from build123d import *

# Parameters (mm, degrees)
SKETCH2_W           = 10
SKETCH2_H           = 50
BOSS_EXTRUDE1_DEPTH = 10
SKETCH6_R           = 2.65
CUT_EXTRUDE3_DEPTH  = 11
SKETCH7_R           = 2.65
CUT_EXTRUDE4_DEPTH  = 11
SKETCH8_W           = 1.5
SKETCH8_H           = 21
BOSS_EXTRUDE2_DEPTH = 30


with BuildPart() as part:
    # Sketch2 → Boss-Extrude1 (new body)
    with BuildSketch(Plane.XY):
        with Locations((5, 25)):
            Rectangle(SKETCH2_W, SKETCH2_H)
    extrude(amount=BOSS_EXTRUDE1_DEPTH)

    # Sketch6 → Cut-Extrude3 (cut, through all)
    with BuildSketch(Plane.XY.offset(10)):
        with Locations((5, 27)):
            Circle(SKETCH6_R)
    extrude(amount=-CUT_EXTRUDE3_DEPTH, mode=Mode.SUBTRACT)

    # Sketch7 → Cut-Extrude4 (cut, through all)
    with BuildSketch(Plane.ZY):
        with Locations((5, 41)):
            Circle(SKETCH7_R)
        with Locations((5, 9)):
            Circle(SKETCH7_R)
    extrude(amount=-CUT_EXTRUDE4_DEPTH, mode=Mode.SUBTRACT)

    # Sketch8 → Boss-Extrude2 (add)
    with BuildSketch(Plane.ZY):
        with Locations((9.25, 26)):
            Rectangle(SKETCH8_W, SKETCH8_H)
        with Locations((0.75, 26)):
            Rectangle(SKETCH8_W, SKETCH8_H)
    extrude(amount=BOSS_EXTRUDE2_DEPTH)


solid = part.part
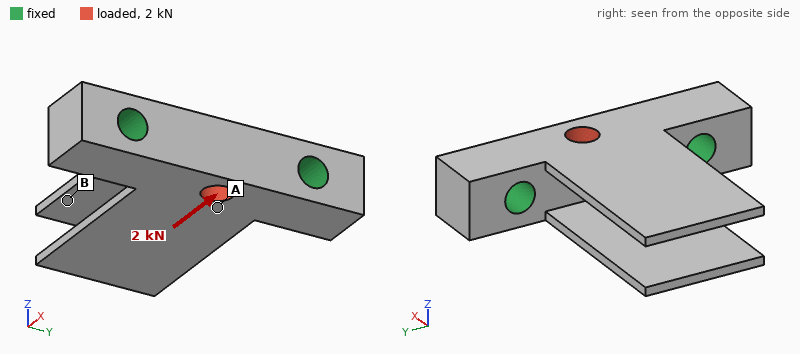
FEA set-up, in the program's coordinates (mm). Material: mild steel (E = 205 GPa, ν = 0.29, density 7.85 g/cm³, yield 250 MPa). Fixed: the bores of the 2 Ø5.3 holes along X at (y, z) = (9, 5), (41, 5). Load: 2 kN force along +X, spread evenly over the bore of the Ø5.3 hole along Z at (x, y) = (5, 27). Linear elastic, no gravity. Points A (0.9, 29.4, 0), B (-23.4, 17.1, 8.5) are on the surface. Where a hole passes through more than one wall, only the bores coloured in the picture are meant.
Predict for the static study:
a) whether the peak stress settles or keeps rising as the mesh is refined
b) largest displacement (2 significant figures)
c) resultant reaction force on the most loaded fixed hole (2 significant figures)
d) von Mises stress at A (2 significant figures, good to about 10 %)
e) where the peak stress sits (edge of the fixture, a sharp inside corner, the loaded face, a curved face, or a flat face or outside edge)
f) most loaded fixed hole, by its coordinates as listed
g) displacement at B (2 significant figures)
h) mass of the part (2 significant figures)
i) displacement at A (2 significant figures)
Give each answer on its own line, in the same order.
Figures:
keeps rising
3.0 µm
1.2 kN
18 MPa
edge of the fixture
(41, 5)
1.9 µm
49 g
2.0 µm
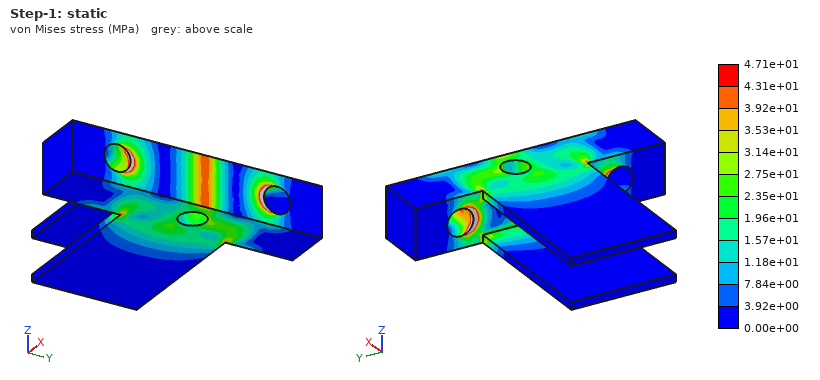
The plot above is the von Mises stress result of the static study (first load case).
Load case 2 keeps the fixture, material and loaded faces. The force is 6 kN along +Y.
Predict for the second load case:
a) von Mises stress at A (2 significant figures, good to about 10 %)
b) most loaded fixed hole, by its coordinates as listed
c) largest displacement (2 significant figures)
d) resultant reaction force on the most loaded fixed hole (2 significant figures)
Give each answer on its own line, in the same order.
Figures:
20 MPa
(41, 5)
2.2 µm
3.3 kN
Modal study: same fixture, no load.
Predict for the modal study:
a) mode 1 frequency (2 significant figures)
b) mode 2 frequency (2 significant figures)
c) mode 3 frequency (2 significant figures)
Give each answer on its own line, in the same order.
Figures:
1300 Hz
1300 Hz
4300 Hz
